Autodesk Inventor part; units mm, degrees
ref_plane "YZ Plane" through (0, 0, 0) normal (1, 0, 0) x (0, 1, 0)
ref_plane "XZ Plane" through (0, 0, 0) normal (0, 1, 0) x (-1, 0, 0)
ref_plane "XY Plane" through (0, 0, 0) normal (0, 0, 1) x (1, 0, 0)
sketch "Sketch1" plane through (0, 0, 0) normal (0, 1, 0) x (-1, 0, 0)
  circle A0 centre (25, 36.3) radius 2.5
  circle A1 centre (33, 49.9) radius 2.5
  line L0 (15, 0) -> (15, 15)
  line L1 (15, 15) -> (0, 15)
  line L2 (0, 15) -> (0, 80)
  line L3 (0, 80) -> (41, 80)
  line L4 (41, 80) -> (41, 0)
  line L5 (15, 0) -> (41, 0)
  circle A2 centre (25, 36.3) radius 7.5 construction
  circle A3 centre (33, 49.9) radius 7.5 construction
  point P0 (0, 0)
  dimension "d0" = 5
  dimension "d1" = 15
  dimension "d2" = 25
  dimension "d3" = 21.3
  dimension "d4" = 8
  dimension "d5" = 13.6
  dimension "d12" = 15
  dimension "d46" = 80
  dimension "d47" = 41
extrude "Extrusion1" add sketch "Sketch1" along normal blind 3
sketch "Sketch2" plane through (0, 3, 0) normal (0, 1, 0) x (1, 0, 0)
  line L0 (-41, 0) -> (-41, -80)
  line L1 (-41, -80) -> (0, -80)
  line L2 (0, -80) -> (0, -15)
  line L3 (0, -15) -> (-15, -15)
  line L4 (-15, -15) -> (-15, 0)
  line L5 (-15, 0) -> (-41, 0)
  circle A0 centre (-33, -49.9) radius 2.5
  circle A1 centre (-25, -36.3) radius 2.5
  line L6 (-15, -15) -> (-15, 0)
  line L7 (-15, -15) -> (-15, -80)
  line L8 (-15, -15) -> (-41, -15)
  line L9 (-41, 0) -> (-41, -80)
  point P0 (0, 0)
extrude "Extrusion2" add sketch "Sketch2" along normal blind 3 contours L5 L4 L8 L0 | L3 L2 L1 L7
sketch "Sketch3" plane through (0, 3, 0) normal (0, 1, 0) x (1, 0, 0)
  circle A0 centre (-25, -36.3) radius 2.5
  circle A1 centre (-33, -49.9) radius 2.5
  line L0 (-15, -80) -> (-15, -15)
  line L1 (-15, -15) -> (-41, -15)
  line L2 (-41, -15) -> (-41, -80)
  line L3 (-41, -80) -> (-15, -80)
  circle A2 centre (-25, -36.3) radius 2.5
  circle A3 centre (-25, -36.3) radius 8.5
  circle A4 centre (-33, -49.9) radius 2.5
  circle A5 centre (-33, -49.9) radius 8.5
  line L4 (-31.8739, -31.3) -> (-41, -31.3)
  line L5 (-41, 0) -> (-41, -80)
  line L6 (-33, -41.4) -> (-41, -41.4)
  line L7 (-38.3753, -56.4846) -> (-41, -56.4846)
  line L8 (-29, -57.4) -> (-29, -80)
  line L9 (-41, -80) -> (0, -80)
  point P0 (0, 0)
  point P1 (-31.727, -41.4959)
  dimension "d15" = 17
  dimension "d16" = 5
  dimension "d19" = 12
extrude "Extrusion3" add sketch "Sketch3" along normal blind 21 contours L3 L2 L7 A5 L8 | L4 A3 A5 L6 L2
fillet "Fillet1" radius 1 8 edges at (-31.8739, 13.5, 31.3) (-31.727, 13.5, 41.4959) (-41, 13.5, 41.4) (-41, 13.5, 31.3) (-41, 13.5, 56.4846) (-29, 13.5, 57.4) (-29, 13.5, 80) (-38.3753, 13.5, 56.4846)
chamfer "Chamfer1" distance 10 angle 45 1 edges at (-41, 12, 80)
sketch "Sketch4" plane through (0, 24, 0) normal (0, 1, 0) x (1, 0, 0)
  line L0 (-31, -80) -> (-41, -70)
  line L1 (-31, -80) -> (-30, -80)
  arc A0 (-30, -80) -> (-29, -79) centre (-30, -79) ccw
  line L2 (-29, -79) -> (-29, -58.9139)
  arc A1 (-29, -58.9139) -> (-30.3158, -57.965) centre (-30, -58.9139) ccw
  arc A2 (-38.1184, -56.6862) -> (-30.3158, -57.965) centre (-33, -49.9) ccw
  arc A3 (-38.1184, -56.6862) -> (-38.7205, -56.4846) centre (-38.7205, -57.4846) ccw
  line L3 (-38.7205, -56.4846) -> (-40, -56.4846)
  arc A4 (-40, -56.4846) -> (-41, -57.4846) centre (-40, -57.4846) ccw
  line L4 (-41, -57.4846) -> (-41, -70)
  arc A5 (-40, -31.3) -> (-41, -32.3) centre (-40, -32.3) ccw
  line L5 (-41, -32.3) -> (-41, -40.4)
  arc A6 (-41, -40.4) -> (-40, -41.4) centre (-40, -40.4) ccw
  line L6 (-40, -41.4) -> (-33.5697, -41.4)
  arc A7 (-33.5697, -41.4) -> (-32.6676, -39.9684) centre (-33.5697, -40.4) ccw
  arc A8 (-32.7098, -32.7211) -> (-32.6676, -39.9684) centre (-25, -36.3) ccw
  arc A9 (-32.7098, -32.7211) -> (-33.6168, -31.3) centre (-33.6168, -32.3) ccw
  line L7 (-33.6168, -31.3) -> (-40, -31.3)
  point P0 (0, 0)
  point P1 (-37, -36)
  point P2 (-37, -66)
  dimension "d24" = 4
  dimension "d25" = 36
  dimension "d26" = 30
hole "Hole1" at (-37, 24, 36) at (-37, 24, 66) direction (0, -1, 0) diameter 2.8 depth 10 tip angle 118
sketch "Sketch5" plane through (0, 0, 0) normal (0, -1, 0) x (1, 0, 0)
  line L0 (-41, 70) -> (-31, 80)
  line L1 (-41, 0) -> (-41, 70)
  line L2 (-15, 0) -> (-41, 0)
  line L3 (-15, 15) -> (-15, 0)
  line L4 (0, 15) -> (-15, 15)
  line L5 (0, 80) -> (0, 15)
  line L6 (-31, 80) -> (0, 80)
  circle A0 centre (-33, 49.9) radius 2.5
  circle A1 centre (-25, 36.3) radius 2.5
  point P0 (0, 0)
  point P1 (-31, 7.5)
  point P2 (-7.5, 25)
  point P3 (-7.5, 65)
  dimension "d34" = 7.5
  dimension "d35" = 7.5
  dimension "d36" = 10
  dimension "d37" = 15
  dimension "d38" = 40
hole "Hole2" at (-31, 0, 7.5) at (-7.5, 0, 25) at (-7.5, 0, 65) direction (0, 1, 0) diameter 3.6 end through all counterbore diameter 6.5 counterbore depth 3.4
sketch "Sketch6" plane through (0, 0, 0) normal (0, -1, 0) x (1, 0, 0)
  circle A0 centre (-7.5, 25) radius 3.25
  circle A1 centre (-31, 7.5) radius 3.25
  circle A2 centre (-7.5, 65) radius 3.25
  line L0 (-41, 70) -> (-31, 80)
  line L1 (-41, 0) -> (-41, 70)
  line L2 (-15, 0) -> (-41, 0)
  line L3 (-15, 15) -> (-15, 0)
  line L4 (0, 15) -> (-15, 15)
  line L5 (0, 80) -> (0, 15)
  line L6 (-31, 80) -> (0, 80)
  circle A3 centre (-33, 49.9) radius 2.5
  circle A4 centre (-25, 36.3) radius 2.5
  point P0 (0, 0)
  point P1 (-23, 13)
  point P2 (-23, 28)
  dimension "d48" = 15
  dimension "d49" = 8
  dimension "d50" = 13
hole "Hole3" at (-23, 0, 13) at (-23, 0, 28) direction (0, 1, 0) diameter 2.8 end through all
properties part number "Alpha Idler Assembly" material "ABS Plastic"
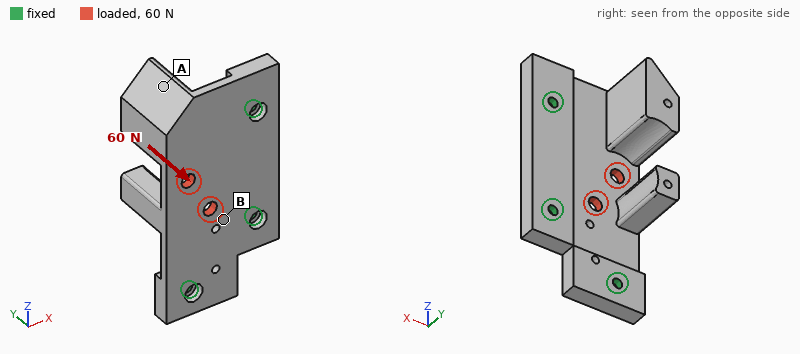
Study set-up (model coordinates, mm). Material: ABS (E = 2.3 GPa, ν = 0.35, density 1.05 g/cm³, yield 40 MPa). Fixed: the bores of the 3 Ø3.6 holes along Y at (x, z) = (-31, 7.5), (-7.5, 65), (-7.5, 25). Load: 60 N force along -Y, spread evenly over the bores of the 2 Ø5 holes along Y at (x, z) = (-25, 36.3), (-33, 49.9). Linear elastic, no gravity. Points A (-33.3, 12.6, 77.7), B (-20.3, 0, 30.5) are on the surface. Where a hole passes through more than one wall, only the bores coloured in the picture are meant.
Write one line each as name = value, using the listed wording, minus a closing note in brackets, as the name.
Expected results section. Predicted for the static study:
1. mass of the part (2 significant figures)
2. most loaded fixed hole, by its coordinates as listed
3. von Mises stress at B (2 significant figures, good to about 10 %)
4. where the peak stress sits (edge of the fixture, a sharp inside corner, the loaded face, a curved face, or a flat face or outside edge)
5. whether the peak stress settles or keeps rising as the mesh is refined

mass of the part = 20 g
most loaded fixed hole, by its coordinates as listed = (-7.5, 65)
von Mises stress at B = 4.4 MPa
where the peak stress sits = edge of the fixture
whether the peak stress settles or keeps rising as the mesh is refined = keeps rising
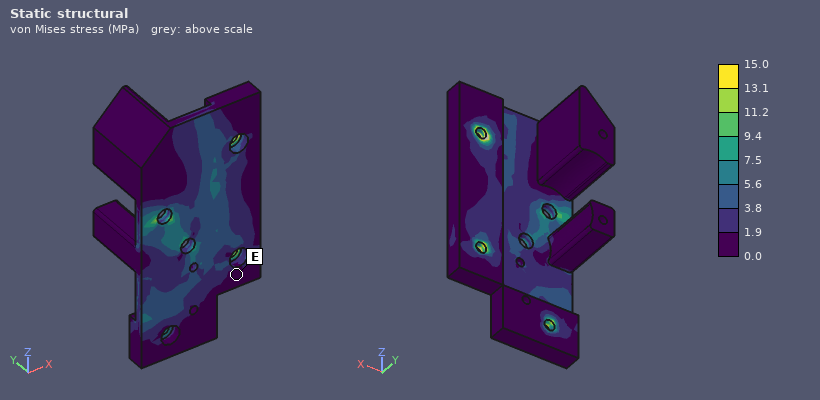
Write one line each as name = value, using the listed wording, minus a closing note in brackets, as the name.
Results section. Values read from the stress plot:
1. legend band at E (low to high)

legend band at E = 0.0 to 1.9 MPa
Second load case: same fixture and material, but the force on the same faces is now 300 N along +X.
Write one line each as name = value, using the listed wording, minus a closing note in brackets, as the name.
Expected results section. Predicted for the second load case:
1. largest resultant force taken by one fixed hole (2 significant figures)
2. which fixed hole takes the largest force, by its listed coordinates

largest resultant force taken by one fixed hole = 140 N
which fixed hole takes the largest force, by its listed coordinates = (-7.5, 25)
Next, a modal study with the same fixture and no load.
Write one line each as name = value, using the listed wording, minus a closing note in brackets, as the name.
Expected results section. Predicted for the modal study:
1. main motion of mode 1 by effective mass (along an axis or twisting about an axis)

main motion of mode 1 by effective mass = along Y
